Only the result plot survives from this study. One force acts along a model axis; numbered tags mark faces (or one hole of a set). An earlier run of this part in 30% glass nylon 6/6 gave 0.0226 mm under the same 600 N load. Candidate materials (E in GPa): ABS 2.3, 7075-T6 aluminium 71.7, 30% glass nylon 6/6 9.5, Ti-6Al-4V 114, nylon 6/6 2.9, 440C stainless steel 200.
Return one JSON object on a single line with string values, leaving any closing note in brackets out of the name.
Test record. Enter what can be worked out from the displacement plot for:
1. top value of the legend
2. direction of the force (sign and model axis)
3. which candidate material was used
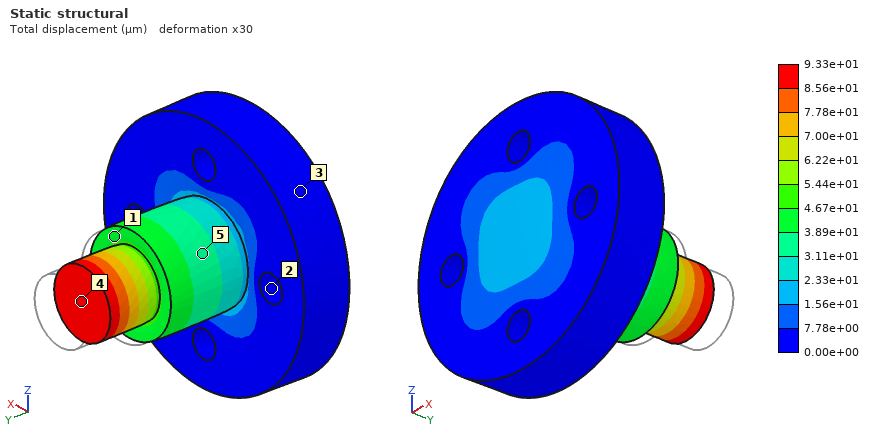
{"top value of the legend": "9.33e+01 µm", "direction of the force": "-Y", "which candidate material was used": "ABS"}
